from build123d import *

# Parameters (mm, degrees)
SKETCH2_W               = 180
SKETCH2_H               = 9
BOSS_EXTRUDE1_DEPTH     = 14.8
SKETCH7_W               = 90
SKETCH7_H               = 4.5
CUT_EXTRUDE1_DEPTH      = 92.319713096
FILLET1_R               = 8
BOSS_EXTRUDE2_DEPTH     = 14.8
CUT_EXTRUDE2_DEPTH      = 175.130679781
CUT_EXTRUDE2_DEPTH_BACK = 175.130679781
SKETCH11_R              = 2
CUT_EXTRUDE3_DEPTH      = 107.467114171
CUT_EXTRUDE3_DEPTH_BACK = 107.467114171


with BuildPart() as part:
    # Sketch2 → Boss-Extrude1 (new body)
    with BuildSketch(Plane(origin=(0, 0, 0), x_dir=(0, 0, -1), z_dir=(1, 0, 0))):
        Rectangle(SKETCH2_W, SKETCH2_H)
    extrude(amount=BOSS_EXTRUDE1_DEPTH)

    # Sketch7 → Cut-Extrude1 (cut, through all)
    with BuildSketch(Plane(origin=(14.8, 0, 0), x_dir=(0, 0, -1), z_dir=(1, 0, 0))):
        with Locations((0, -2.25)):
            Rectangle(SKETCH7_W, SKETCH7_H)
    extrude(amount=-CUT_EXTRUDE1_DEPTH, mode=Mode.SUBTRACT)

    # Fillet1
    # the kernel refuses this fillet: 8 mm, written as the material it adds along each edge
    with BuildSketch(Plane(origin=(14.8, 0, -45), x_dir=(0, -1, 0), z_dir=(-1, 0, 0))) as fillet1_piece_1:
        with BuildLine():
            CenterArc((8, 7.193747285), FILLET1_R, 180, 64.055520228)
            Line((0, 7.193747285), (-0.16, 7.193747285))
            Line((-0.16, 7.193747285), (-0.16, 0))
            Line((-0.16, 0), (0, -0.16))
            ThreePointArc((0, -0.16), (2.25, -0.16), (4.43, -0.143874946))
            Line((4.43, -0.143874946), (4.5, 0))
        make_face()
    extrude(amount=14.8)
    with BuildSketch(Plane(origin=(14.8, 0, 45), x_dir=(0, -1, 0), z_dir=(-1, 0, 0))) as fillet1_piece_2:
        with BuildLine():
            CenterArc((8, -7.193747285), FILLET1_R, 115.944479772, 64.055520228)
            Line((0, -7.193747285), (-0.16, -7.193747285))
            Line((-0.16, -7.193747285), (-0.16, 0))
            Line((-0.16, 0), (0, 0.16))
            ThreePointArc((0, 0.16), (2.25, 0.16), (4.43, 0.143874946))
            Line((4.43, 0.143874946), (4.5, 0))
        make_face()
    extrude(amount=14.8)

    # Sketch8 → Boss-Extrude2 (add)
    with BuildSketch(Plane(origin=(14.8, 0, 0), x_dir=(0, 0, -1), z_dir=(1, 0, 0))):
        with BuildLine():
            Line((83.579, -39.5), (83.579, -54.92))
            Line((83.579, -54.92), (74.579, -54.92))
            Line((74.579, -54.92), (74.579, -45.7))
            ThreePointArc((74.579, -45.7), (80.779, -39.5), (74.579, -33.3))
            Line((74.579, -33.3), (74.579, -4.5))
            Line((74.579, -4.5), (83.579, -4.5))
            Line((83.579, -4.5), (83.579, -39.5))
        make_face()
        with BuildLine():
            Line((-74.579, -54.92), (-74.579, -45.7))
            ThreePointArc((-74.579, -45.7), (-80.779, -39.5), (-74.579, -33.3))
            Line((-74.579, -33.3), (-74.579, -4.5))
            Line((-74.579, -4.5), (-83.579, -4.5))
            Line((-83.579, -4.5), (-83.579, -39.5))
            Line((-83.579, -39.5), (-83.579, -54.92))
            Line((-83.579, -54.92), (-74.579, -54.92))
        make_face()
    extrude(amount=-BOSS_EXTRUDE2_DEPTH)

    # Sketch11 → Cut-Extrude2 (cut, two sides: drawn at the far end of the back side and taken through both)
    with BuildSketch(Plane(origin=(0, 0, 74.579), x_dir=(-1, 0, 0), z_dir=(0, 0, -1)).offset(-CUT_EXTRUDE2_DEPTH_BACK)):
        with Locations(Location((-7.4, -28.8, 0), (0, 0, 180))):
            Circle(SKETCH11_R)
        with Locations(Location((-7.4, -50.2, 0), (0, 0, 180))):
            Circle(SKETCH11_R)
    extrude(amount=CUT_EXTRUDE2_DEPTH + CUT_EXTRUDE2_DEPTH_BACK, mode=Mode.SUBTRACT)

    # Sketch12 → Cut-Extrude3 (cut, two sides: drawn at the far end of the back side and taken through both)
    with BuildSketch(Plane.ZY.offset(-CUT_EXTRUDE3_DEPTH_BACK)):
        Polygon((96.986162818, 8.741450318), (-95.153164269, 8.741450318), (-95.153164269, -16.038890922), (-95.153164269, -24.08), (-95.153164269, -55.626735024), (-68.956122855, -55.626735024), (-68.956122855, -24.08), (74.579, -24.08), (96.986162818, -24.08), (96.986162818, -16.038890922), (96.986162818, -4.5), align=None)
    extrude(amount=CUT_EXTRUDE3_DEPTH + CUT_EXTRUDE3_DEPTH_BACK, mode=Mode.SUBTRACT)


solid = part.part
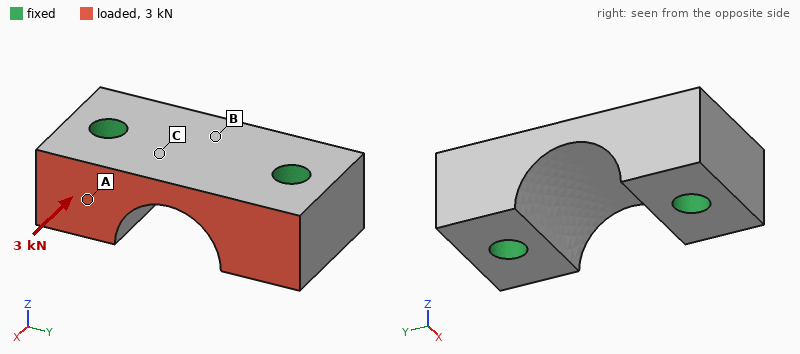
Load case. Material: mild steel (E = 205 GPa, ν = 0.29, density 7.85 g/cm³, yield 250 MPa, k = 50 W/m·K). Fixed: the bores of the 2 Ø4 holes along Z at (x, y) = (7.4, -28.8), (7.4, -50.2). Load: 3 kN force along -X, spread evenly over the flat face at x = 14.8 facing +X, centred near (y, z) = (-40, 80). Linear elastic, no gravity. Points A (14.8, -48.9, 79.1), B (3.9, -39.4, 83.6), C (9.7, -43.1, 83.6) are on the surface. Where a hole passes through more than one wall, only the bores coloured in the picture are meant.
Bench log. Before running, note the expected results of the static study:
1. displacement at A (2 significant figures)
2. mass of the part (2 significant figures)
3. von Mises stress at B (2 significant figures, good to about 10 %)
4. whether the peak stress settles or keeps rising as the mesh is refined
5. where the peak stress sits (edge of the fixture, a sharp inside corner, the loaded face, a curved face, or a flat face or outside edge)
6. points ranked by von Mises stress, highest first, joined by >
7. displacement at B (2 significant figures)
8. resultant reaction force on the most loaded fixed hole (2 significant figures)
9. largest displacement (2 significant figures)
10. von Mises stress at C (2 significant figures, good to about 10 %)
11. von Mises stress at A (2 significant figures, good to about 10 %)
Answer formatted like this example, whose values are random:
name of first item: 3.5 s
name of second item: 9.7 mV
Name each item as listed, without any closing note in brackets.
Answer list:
displacement at A: 0.57 µm
mass of the part: 23 g
von Mises stress at B: 4.6 MPa
whether the peak stress settles or keeps rising as the mesh is refined: keeps rising
where the peak stress sits: edge of the fixture
points ranked by von Mises stress, highest first, joined by >: A > C > B
displacement at B: 0.76 µm
resultant reaction force on the most loaded fixed hole: 1.5 kN
largest displacement: 1.3 µm
von Mises stress at C: 12 MPa
von Mises stress at A: 18 MPa
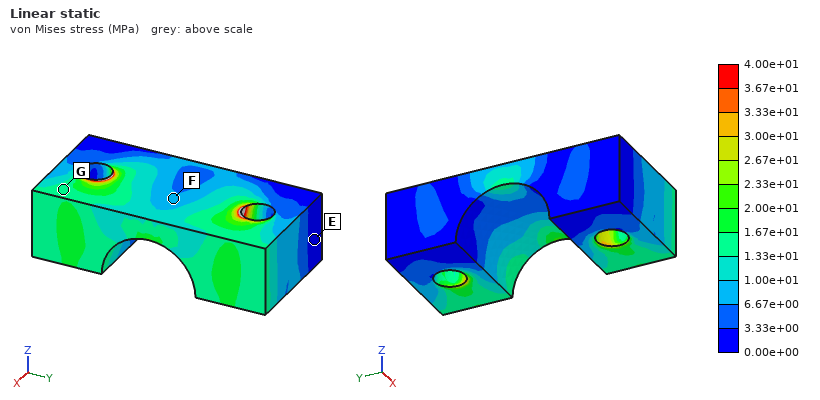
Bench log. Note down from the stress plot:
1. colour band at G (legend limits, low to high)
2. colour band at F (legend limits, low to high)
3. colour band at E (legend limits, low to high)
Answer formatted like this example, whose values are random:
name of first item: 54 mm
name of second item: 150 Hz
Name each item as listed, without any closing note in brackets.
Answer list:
colour band at G: 1.33e+01 to 1.67e+01 MPa
colour band at F: 6.67e+00 to 1.00e+01 MPa
colour band at E: 0.00e+00 to 3.33e+00 MPa
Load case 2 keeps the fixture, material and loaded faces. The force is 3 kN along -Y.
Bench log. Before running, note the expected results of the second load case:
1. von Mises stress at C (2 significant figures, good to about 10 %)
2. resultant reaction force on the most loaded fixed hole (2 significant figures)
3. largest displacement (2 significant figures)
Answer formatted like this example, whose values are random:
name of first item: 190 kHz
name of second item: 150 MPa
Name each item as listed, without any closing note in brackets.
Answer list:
von Mises stress at C: 26 MPa
resultant reaction force on the most loaded fixed hole: 1.6 kN
largest displacement: 3.0 µm
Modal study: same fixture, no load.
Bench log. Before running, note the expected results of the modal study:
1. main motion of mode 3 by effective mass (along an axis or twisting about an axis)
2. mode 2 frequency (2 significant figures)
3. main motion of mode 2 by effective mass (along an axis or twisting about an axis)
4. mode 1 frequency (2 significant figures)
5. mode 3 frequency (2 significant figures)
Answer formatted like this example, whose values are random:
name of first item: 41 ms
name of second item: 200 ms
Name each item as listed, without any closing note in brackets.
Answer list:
main motion of mode 3 by effective mass: twisting about Y
mode 2 frequency: 66 kHz
main motion of mode 2 by effective mass: along Z
mode 1 frequency: 57 kHz
mode 3 frequency: 75 kHz
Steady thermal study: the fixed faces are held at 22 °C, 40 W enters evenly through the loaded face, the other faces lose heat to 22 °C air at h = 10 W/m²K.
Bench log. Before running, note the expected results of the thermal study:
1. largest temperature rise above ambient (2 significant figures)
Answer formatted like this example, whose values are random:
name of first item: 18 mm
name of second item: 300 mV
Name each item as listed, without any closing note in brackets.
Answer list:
largest temperature rise above ambient: 31 K
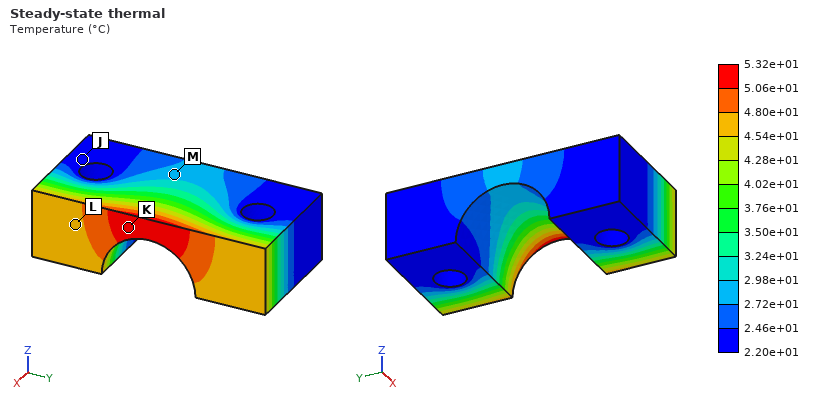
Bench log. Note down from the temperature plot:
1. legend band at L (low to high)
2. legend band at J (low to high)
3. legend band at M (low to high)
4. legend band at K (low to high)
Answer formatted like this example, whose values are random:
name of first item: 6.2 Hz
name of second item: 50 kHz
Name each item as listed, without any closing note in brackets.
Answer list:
legend band at L: 4.54e+01 to 4.80e+01 °C
legend band at J: 2.20e+01 to 2.46e+01 °C
legend band at M: 2.72e+01 to 2.98e+01 °C
legend band at K: 5.06e+01 to 5.32e+01 °C
